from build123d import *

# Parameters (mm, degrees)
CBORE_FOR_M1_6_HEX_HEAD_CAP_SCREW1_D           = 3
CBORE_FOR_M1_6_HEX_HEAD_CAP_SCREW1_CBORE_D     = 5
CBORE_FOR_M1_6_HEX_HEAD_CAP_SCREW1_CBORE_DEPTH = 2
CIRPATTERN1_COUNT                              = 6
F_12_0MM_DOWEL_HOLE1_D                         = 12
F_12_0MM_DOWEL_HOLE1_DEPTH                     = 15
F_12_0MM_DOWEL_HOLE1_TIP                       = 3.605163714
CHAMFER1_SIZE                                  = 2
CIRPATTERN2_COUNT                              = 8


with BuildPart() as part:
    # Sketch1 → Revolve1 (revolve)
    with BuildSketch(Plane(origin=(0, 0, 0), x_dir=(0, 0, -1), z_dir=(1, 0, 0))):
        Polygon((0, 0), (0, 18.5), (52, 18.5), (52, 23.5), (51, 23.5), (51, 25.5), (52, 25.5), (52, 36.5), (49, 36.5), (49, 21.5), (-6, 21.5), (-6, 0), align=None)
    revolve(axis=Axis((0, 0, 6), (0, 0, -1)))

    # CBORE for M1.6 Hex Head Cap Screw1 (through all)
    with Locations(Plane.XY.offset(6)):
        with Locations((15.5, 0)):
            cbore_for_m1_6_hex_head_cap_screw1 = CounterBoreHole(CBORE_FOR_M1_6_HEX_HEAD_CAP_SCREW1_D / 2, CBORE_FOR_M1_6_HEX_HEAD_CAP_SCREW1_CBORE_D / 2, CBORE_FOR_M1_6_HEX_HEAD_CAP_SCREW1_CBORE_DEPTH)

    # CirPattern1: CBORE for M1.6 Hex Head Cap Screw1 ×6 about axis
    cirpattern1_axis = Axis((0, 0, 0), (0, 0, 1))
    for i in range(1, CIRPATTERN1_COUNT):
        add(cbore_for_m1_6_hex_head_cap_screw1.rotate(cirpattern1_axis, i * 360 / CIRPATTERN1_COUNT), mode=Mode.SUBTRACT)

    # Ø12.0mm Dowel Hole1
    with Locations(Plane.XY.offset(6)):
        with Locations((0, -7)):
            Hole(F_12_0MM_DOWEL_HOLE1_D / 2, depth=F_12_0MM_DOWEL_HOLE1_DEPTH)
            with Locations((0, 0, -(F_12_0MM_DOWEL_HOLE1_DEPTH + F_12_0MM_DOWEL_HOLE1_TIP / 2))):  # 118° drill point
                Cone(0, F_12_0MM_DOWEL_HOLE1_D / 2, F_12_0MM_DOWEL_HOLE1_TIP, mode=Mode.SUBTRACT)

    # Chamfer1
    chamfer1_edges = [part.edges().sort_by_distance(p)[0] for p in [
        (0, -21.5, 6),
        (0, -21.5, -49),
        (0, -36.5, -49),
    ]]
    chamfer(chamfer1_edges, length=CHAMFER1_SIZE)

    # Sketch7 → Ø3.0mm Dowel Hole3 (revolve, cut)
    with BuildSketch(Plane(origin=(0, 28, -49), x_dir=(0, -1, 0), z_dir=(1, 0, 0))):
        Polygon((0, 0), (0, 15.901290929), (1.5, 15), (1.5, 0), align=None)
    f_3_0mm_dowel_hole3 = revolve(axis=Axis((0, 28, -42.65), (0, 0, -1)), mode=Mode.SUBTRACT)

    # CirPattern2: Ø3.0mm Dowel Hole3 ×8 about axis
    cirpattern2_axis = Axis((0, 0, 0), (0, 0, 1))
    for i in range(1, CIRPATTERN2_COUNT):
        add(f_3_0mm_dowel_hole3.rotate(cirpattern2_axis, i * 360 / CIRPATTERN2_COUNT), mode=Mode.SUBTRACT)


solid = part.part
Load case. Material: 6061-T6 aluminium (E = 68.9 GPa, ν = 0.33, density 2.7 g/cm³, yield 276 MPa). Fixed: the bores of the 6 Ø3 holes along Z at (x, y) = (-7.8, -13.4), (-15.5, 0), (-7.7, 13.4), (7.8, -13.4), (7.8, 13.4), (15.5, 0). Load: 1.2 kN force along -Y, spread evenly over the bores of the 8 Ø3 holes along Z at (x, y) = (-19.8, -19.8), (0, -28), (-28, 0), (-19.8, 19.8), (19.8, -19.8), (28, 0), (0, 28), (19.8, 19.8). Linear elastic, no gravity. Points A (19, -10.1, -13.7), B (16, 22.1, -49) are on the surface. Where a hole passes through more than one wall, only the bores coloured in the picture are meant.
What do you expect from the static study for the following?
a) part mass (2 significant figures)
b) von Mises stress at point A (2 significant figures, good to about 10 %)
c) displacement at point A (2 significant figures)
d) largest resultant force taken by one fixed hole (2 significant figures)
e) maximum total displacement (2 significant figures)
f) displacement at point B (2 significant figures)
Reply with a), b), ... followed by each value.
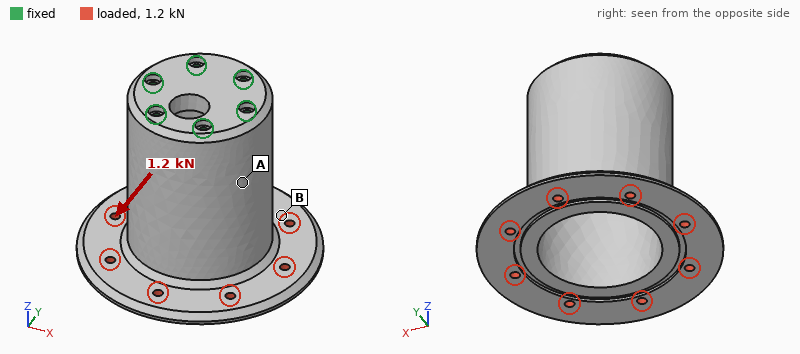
a) 93 g
b) 11 MPa
c) 13 µm
d) 1.0 kN
e) 54 µm
f) 45 µm
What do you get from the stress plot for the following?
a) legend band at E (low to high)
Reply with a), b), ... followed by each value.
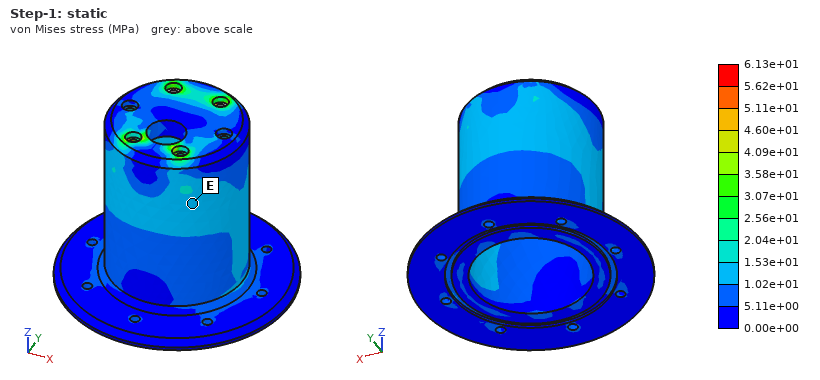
a) 1.02e+01 to 1.53e+01 MPa
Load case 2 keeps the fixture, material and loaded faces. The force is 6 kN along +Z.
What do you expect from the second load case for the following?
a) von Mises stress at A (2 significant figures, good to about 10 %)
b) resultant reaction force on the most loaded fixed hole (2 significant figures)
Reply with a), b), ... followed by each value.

a) 18 MPa
b) 1.0 kN
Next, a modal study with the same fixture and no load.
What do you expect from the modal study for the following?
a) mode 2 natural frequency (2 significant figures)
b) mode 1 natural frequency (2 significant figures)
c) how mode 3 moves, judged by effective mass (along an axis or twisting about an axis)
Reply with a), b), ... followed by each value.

a) 4000 Hz
b) 4000 Hz
c) along Z
